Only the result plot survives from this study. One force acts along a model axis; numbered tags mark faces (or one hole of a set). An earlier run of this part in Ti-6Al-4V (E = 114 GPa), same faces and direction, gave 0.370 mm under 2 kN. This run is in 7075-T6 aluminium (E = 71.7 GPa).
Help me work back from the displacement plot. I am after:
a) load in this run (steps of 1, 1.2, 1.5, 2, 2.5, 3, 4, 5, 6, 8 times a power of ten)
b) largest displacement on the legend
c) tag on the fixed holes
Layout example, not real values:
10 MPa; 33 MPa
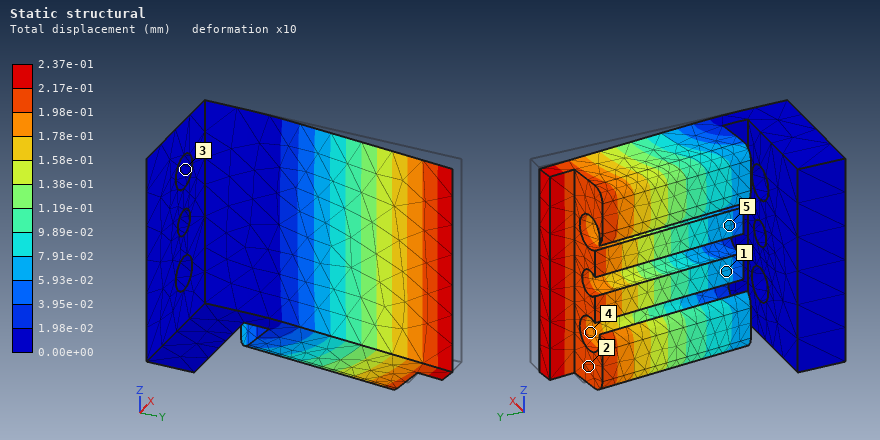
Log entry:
800 N; 2.37e-01 mm; 3
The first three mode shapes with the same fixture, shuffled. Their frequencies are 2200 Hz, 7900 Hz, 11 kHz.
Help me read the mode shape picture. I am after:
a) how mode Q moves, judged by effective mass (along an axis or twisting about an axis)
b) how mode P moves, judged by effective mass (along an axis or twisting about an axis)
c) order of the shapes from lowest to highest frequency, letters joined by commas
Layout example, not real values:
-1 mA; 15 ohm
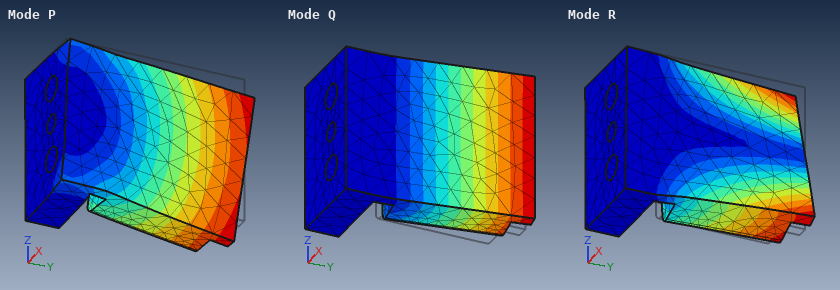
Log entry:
along X; along Z; Q, R, P
